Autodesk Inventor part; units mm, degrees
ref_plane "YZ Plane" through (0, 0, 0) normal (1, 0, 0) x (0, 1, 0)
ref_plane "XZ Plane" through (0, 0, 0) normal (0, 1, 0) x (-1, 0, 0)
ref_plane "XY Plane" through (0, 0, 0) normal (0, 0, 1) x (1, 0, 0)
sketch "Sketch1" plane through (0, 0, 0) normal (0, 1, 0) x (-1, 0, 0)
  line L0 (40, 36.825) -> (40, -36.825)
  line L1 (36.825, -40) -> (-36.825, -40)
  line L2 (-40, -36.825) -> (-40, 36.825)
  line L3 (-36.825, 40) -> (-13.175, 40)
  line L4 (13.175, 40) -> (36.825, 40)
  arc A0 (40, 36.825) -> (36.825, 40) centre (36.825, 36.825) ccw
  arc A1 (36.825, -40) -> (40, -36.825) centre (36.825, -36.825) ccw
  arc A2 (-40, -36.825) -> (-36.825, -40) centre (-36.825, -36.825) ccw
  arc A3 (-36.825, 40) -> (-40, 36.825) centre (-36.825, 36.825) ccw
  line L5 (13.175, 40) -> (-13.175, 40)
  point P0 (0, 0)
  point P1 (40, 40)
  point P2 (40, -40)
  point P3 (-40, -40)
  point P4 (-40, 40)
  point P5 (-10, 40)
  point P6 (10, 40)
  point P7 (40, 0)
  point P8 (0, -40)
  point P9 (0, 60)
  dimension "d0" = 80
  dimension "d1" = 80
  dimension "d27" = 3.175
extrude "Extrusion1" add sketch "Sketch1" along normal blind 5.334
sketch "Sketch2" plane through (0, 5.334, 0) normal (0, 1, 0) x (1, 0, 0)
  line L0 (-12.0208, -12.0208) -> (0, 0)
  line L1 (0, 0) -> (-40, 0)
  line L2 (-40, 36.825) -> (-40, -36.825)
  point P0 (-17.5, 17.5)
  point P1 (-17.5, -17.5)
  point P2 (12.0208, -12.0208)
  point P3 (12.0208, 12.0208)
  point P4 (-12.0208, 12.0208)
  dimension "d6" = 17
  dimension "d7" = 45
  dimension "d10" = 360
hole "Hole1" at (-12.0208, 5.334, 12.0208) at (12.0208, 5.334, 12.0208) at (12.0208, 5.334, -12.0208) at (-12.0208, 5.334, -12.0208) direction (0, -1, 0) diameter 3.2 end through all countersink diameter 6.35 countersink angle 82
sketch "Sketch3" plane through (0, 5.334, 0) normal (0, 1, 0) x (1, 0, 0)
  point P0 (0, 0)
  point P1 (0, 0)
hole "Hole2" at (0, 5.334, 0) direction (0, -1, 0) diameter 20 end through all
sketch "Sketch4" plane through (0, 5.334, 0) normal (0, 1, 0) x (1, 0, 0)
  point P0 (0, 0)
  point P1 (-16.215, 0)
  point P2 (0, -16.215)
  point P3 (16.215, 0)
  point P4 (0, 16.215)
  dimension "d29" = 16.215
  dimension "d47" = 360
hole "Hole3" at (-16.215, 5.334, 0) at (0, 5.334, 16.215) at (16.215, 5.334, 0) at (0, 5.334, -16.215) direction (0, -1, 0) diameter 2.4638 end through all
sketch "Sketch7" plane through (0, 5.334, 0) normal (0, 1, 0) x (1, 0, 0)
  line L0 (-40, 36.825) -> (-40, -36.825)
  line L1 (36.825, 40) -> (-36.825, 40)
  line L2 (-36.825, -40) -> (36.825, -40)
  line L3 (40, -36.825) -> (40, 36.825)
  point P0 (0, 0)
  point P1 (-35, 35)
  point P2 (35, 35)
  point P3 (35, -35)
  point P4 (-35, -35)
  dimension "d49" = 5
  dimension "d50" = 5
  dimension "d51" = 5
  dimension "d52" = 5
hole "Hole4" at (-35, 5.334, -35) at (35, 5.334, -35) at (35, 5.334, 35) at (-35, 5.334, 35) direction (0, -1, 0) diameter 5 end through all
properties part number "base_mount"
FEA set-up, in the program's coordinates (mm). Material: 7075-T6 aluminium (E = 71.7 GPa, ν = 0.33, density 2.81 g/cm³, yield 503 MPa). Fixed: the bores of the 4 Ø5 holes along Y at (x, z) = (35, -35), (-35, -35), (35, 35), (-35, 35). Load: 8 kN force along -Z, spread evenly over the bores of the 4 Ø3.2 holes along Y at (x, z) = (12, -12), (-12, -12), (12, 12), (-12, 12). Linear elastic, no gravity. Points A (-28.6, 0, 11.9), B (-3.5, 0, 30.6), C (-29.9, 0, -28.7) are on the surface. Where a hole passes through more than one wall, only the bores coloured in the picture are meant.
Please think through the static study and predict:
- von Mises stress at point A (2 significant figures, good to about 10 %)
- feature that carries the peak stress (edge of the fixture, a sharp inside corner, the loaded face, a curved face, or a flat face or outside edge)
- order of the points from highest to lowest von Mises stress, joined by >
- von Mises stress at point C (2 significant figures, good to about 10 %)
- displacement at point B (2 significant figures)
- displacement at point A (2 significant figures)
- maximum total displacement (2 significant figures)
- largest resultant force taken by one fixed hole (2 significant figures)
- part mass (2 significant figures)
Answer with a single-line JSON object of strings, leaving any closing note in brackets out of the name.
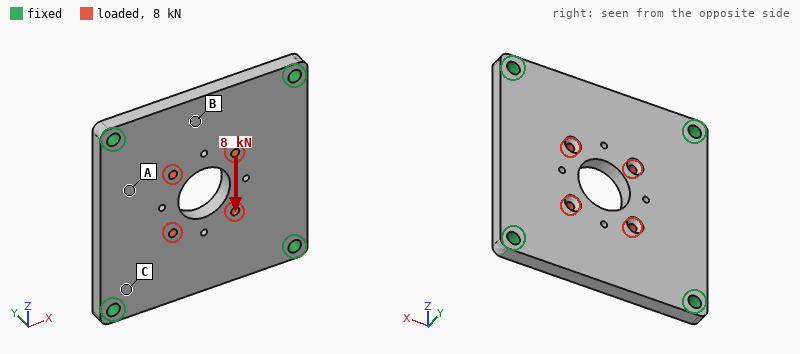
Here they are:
{"von Mises stress at point A": "16 MPa", "feature that carries the peak stress": "the loaded face", "order of the points from highest to lowest von Mises stress, joined by >": "C > A > B", "von Mises stress at point C": "30 MPa", "displacement at point B": "14 µm", "displacement at point A": "7.0 µm", "maximum total displacement": "17 µm", "largest resultant force taken by one fixed hole": "2.2 kN", "part mass": "89 g"}
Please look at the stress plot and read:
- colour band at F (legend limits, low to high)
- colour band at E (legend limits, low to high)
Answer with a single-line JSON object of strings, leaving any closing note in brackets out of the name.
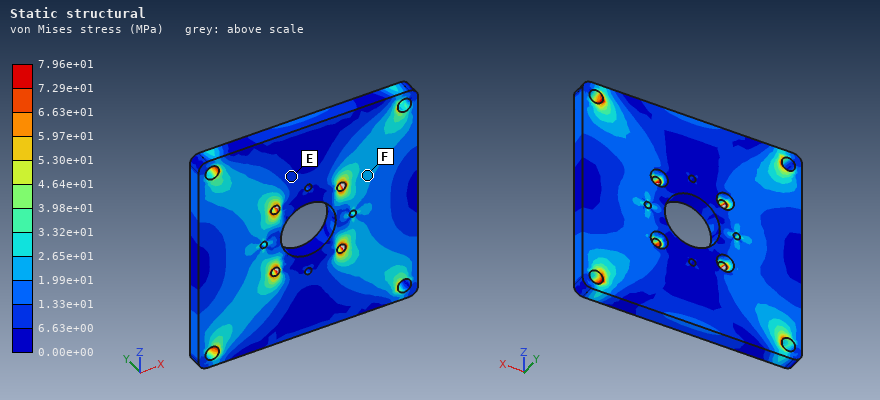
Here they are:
{"colour band at F": "1.99e+01 to 2.65e+01 MPa", "colour band at E": "6.63e+00 to 1.33e+01 MPa"}
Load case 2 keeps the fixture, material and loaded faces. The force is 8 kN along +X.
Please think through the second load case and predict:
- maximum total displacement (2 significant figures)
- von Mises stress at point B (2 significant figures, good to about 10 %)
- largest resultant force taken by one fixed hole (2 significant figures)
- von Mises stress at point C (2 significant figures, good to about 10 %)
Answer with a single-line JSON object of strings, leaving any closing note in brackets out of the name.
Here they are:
{"maximum total displacement": "17 µm", "von Mises stress at point B": "13 MPa", "largest resultant force taken by one fixed hole": "2.2 kN", "von Mises stress at point C": "28 MPa"}
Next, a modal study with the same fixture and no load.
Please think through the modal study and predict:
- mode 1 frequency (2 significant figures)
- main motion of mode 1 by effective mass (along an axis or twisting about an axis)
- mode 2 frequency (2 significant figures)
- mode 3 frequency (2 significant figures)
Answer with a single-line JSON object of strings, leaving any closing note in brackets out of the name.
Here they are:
{"mode 1 frequency": "3600 Hz", "main motion of mode 1 by effective mass": "along Y", "mode 2 frequency": "6100 Hz", "mode 3 frequency": "6100 Hz"}
